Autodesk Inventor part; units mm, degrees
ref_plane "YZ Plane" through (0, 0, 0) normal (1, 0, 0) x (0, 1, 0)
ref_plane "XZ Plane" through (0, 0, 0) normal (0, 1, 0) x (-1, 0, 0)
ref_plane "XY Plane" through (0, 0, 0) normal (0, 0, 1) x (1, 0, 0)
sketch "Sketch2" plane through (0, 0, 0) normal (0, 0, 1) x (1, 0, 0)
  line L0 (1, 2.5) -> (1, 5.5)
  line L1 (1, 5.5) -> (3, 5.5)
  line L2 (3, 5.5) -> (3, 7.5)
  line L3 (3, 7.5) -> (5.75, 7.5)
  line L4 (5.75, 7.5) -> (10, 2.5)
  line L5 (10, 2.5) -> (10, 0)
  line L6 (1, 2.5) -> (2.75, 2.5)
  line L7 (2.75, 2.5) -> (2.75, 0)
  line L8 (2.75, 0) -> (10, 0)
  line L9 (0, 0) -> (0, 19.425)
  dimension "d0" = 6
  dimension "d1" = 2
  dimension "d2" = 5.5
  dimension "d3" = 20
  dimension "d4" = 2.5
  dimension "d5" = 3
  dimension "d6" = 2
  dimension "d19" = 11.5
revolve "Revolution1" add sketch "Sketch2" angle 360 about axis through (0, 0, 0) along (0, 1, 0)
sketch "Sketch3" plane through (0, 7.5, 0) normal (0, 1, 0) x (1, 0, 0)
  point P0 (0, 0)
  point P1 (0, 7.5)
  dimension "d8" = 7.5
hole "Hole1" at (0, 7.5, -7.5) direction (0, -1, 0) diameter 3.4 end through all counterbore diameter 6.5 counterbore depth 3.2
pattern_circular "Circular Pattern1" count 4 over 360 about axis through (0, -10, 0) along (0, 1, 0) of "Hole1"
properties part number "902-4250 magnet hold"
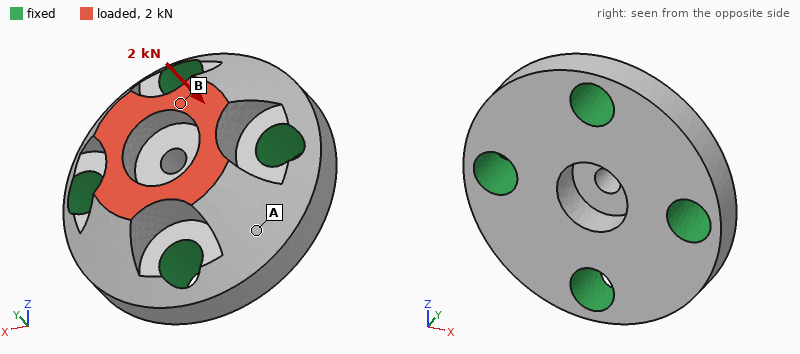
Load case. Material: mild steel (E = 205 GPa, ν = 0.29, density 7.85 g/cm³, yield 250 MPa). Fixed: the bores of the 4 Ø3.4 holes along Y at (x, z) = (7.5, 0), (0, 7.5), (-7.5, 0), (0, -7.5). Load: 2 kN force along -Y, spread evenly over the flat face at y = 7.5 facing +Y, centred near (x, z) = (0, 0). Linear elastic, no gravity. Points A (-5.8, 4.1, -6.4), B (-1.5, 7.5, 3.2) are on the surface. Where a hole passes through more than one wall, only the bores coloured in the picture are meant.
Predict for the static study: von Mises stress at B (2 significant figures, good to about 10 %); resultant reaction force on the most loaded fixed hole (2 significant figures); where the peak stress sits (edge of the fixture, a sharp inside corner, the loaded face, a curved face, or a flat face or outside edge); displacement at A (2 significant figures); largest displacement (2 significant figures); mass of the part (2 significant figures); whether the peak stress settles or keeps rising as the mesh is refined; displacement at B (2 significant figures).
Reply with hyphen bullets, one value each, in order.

- 29 MPa
- 530 N
- edge of the fixture
- 0.32 µm
- 1.2 µm
- 11 g
- keeps rising
- 1.2 µm
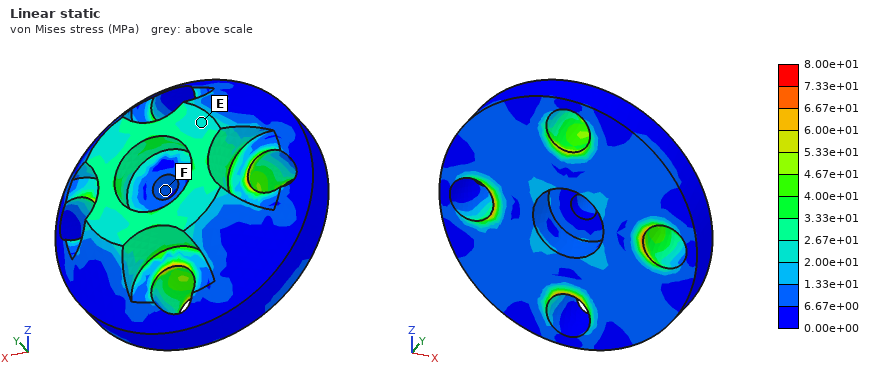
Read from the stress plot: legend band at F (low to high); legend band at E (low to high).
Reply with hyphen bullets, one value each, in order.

- 6.67e+00 to 1.33e+01 MPa
- 2.00e+01 to 2.67e+01 MPa
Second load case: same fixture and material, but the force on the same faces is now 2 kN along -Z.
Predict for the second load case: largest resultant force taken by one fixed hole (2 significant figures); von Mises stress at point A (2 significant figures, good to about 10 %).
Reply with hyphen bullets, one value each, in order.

- 870 N
- 18 MPa
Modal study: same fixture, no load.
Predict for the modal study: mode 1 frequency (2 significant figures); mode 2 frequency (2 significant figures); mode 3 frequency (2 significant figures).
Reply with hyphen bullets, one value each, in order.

- 110 kHz
- 110 kHz
- 120 kHz
